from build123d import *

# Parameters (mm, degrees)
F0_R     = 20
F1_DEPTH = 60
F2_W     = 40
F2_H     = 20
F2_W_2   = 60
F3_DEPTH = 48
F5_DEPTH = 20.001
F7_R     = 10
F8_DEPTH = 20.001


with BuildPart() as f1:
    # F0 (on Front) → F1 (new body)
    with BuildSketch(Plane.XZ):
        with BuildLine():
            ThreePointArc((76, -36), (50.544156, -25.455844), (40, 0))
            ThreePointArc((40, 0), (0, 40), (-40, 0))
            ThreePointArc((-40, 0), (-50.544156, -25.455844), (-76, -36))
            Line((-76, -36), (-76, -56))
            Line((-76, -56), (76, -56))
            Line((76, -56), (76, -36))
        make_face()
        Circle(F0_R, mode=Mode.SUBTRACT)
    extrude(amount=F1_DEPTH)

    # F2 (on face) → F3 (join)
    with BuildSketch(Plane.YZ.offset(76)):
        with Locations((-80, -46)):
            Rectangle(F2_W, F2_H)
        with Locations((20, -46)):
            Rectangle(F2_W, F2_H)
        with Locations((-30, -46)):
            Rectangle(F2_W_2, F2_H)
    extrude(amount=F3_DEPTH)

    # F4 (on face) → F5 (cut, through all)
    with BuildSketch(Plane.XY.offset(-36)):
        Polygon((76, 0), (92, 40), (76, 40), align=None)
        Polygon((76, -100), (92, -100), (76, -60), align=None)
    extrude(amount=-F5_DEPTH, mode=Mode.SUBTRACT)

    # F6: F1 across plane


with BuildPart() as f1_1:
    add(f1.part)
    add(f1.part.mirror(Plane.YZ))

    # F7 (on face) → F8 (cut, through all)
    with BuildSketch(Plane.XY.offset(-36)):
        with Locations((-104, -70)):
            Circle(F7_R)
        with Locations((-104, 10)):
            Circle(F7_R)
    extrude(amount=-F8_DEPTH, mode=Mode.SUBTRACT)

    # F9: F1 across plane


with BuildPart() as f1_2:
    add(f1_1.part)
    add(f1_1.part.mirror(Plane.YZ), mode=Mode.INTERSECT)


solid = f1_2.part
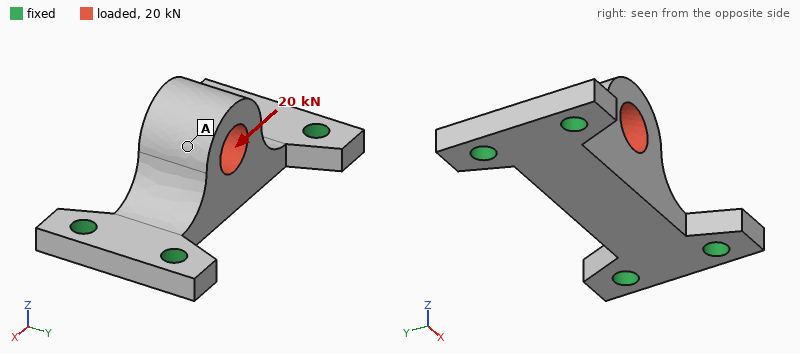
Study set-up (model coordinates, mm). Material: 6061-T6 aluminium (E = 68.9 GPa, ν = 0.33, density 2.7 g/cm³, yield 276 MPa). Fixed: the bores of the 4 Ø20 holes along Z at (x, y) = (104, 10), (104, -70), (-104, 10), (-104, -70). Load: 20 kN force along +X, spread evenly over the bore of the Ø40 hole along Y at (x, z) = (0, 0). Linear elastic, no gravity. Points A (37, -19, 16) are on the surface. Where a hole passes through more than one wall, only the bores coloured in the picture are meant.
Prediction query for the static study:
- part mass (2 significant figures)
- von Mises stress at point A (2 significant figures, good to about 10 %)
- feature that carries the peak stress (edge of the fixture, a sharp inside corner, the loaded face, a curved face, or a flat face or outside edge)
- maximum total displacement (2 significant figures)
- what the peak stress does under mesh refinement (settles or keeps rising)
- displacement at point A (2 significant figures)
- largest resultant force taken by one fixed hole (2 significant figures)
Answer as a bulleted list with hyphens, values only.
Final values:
- 1.8 kg
- 4.5 MPa
- edge of the fixture
- 54 µm
- keeps rising
- 47 µm
- 6.1 kN
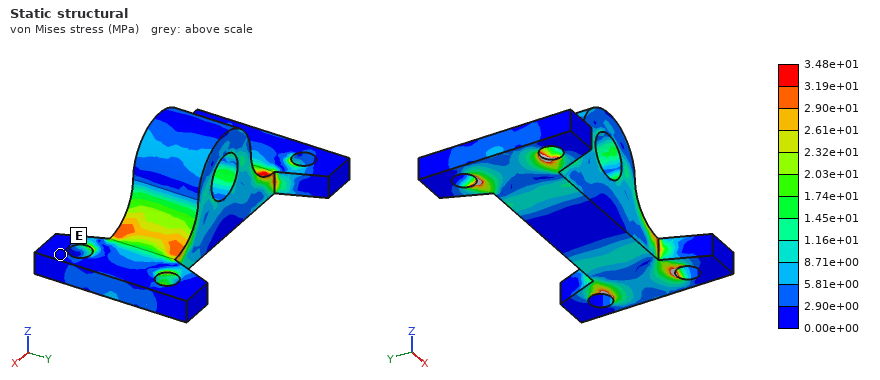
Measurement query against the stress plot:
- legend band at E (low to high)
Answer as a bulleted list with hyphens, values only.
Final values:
- 0.00e+00 to 2.90e+00 MPa
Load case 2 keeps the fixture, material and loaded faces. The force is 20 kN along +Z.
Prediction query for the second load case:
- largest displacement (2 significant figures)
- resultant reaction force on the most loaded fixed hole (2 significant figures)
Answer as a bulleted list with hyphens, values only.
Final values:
- 84 µm
- 6.5 kN
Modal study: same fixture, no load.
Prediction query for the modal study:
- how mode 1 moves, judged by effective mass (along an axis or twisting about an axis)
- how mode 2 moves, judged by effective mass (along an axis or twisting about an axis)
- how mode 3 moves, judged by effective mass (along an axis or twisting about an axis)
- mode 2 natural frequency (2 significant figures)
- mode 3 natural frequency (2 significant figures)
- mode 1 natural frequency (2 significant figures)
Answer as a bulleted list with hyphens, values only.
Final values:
- along Y
- along Z
- along X
- 2400 Hz
- 3900 Hz
- 1700 Hz
